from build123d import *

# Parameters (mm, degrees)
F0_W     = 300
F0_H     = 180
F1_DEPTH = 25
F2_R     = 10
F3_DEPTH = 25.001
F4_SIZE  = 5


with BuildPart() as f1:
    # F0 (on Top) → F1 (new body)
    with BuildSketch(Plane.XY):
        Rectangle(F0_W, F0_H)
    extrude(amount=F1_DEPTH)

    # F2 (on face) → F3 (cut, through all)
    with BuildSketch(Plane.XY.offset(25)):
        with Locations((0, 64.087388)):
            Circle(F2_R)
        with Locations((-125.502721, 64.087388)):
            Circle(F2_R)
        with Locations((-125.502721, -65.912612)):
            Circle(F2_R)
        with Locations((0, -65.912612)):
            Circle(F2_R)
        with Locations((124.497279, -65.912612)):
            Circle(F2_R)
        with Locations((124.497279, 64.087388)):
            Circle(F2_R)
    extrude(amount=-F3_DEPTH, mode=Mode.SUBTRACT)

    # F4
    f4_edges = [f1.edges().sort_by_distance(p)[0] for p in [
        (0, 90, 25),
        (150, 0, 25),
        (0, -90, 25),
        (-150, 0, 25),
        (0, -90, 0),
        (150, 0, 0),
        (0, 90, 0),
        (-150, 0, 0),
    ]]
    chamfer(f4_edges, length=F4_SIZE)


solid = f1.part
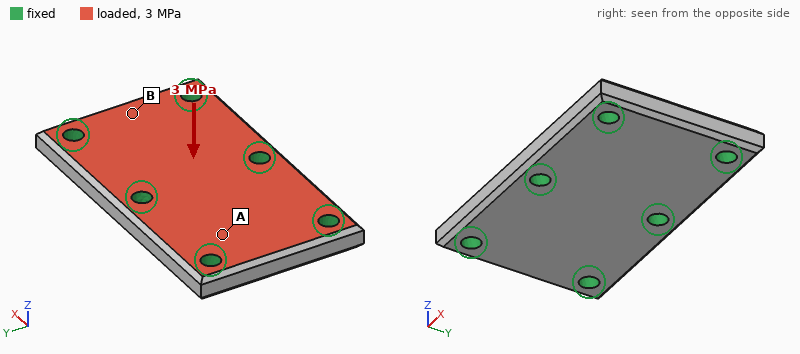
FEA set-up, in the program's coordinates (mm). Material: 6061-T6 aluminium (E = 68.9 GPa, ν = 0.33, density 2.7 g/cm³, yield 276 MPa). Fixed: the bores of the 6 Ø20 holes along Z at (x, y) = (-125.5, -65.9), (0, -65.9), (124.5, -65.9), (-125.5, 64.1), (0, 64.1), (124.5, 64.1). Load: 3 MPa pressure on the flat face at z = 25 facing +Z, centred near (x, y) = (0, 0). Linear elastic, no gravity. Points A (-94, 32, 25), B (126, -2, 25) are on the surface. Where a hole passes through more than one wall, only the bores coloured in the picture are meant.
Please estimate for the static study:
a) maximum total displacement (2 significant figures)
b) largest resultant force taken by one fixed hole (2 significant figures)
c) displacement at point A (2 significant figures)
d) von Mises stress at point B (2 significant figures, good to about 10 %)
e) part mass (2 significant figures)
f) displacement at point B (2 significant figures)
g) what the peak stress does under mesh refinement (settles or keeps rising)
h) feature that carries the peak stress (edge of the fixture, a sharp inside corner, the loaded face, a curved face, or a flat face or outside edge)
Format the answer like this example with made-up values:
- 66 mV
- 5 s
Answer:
- 58 µm
- 32 kN
- 39 µm
- 18 MPa
- 3.5 kg
- 34 µm
- keeps rising
- edge of the fixture
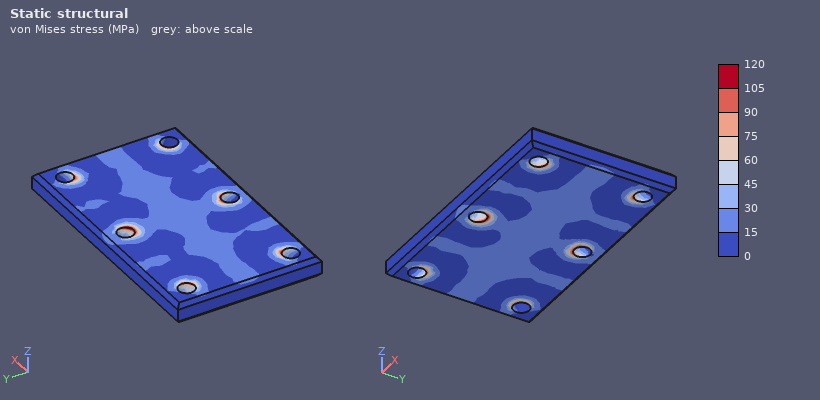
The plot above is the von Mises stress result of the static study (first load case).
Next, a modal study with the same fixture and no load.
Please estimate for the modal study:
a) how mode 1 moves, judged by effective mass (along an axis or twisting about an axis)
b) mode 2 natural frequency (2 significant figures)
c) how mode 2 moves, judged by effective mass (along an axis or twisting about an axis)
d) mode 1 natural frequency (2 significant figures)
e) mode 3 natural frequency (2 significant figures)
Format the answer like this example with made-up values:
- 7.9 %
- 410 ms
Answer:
- along Z
- 5500 Hz
- twisting about Y
- 5200 Hz
- 7700 Hz
